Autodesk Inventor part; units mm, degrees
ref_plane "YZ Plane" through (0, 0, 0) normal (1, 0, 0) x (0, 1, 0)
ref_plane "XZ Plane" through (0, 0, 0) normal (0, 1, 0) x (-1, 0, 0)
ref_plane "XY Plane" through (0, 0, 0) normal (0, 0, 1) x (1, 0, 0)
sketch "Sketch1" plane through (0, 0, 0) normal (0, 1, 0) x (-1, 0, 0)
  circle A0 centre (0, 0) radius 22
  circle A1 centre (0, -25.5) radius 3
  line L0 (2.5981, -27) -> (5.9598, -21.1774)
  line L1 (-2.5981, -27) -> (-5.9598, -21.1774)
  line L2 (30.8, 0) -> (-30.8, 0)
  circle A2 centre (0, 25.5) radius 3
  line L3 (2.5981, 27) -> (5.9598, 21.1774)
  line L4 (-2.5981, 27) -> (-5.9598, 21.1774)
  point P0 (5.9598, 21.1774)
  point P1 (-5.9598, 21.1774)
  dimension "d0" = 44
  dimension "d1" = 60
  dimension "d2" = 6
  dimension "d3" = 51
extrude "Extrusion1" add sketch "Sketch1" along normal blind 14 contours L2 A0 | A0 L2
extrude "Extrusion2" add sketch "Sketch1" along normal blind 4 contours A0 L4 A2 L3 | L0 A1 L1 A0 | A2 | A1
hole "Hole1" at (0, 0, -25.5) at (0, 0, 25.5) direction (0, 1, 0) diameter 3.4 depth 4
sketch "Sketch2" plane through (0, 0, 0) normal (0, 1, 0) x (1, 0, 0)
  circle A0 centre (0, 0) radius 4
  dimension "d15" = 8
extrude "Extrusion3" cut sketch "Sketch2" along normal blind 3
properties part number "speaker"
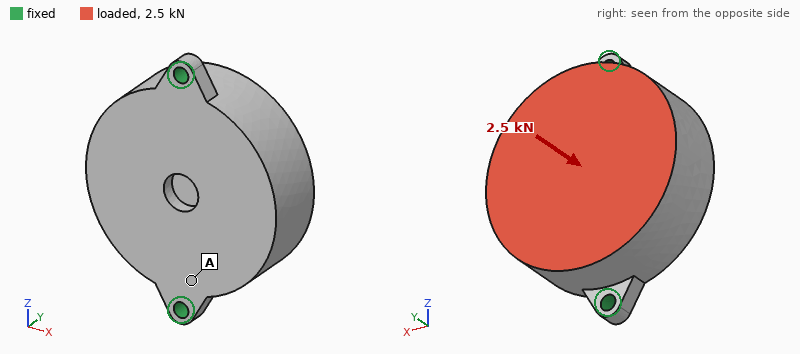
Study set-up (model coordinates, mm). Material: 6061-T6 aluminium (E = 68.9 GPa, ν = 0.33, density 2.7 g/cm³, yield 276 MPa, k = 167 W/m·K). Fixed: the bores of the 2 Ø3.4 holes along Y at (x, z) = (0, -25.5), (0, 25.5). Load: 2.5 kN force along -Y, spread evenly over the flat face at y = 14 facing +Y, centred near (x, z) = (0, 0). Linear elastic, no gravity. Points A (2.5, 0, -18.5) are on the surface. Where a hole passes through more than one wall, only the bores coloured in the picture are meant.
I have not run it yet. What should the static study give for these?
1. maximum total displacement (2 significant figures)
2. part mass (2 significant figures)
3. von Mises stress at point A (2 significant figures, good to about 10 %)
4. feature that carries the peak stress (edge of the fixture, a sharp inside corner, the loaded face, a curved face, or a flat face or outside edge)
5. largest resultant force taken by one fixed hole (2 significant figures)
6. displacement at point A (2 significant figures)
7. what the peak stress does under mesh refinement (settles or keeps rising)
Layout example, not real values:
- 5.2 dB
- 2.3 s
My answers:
- 20 µm
- 58 g
- 20 MPa
- edge of the fixture
- 1.5 kN
- 12 µm
- keeps rising
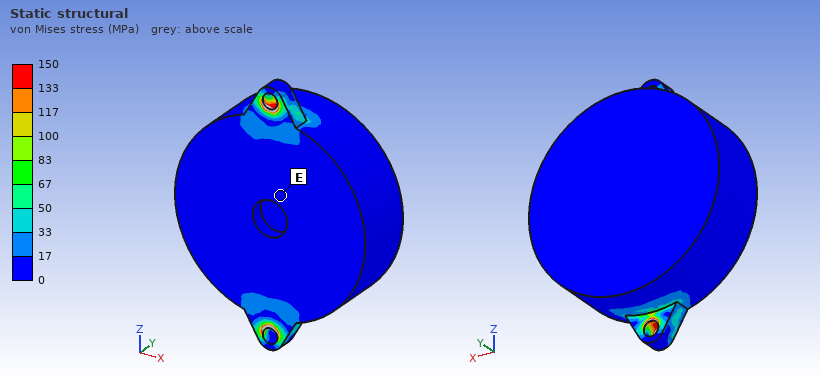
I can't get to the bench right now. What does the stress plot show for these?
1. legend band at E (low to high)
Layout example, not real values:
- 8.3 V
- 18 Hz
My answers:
- 0 to 17 MPa
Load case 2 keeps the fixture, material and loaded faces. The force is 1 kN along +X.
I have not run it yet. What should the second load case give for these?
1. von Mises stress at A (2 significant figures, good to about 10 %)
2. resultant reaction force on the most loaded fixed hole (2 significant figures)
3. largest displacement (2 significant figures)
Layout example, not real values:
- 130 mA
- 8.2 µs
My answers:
- 38 MPa
- 500 N
- 0.14 mm
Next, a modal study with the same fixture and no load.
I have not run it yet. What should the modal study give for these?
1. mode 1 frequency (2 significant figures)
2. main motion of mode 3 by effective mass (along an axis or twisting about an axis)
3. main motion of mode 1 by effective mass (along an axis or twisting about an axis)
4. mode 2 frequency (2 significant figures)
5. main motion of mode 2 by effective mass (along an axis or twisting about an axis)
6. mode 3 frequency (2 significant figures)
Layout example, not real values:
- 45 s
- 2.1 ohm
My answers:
- 2400 Hz
- along X
- along X
- 8300 Hz
- along Y
- 12 kHz
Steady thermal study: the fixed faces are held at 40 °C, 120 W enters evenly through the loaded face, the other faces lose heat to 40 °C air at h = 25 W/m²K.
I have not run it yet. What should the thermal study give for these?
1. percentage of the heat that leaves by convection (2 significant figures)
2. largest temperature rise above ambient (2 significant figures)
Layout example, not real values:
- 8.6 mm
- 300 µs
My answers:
- 4.3 %
- 65 K
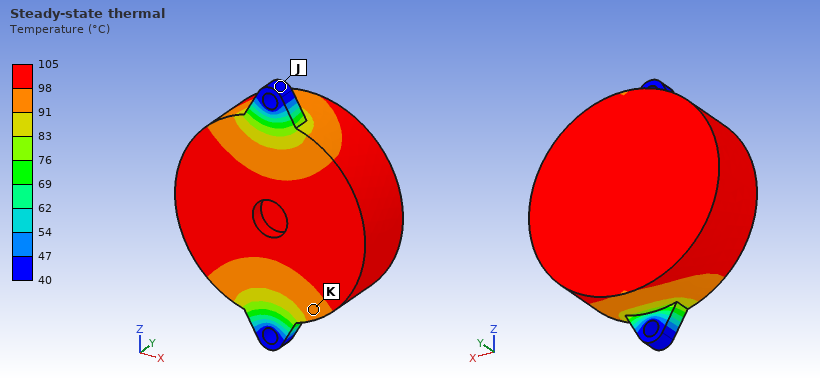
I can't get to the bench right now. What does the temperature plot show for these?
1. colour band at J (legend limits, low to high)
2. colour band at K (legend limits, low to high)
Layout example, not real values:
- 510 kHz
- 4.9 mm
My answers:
- 40 to 47 °C
- 91 to 98 °C
